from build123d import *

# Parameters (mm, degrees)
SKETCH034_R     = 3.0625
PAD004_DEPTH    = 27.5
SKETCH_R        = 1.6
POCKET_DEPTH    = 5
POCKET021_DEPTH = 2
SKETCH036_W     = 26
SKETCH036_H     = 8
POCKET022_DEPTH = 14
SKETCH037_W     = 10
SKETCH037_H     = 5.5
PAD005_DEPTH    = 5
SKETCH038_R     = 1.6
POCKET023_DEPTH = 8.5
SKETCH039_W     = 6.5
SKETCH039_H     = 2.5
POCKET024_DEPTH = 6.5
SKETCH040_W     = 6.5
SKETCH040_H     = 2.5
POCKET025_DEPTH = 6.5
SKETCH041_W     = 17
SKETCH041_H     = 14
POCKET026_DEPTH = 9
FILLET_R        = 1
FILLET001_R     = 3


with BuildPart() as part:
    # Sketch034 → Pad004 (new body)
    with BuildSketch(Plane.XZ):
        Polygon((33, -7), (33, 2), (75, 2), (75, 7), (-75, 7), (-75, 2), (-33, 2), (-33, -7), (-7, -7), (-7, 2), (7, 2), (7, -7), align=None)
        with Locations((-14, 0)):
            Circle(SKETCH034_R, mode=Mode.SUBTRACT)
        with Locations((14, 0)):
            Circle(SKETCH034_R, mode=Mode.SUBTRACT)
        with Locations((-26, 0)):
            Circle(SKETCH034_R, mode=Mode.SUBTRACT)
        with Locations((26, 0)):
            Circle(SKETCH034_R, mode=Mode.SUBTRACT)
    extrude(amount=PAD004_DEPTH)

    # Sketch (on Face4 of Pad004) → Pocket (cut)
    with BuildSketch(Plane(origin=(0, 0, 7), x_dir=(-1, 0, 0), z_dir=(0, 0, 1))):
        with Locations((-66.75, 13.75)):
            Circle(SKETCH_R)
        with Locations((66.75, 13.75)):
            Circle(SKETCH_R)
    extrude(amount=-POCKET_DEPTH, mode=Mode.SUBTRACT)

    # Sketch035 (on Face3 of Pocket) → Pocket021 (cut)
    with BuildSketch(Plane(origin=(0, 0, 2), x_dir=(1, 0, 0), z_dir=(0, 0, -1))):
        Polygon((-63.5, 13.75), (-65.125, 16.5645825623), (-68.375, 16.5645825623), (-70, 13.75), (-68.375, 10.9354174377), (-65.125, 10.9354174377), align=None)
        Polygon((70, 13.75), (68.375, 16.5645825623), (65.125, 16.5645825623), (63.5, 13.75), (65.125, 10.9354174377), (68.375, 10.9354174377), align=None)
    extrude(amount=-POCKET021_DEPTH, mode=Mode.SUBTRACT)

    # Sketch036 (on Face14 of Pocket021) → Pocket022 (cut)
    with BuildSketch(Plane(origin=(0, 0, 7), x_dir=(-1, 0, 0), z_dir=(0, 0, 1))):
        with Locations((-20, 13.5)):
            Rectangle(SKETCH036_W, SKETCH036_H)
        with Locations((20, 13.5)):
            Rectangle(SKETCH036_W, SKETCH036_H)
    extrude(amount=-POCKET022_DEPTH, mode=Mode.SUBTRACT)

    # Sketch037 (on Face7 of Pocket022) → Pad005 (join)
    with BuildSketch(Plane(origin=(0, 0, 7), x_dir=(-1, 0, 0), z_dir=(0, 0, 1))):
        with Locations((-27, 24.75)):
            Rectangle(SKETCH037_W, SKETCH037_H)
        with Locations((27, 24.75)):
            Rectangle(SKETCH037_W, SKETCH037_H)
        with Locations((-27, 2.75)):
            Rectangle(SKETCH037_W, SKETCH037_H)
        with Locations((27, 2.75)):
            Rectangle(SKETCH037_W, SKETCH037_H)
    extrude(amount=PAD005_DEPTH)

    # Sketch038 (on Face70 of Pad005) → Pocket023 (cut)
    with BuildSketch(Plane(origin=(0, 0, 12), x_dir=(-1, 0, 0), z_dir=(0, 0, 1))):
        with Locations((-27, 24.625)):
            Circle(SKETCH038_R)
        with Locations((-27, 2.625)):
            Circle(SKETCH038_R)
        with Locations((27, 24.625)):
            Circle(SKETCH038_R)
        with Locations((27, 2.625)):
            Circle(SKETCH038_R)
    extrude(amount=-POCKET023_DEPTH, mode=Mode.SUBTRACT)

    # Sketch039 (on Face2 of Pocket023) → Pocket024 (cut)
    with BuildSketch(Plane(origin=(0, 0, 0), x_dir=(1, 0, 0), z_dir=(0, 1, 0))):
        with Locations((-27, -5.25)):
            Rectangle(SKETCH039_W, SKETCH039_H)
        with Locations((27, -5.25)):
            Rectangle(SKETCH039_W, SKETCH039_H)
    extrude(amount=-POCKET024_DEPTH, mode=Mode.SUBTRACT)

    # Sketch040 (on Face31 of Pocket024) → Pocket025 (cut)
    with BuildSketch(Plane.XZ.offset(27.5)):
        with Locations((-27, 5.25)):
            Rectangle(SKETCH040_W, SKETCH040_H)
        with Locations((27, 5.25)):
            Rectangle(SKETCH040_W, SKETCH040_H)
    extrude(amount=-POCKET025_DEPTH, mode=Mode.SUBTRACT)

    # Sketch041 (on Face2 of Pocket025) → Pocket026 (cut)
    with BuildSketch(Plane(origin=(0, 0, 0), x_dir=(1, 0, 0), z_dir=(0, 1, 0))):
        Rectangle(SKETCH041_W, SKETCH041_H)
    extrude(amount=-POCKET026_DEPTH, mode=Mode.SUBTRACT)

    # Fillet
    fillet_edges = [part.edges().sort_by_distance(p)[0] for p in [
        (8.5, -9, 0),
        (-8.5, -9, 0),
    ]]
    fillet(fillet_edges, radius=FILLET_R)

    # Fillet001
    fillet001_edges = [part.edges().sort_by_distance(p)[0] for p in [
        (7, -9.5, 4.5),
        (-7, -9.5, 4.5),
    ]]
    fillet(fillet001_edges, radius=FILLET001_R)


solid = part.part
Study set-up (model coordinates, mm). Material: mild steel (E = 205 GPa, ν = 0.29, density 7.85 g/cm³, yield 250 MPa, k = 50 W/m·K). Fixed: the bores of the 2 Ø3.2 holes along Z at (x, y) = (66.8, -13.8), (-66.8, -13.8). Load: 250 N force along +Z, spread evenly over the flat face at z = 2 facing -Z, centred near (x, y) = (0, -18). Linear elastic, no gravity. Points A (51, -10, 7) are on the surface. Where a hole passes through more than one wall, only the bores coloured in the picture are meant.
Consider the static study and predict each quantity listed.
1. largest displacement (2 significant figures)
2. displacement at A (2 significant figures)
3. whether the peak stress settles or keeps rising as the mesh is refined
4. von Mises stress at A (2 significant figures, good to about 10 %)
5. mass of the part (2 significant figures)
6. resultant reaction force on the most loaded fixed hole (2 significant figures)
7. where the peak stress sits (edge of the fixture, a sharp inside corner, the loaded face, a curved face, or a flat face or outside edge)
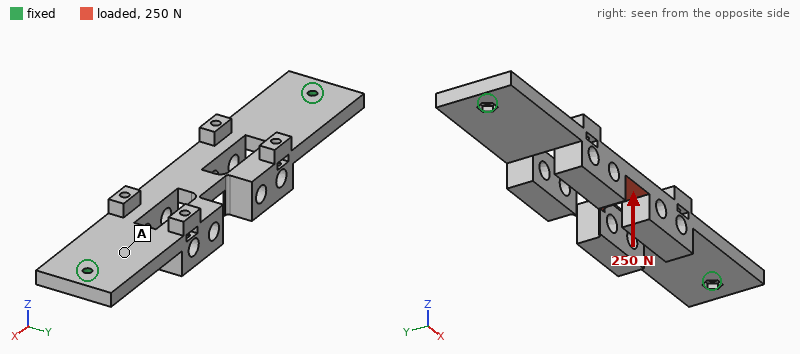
86 µm
16 µm
keeps rising
14 MPa
190 g
230 N
edge of the fixture
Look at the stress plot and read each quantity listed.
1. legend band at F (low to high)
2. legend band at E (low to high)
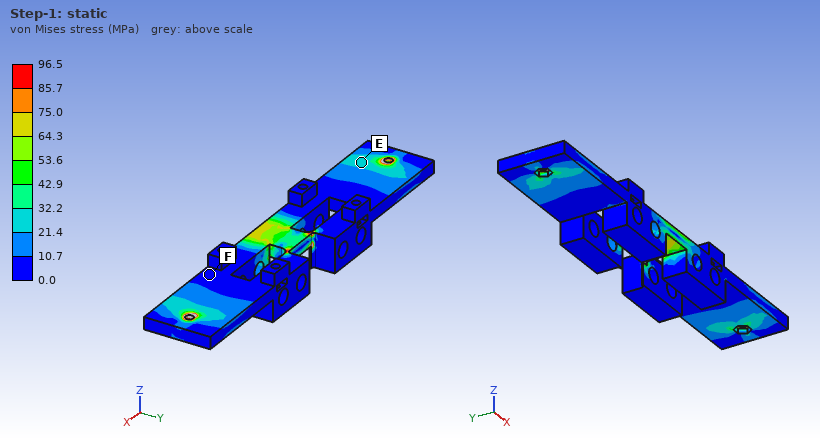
0.0 to 10.7 MPa
21.4 to 32.2 MPa
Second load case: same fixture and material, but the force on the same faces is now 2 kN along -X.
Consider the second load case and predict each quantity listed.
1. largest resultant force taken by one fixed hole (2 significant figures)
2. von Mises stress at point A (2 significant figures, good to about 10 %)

1.0 kN
8.2 MPa
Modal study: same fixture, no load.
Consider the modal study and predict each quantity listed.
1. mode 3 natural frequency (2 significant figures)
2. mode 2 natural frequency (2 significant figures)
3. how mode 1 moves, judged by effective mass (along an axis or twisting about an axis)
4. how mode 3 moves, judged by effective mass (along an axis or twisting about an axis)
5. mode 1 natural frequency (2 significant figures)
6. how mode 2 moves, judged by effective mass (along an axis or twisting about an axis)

2700 Hz
2000 Hz
along Z
along Y
1000 Hz
along Y
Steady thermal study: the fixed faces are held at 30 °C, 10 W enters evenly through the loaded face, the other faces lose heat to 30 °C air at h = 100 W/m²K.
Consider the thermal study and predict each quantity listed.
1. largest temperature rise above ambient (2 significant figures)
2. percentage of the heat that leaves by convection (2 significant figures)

26 K
88 %
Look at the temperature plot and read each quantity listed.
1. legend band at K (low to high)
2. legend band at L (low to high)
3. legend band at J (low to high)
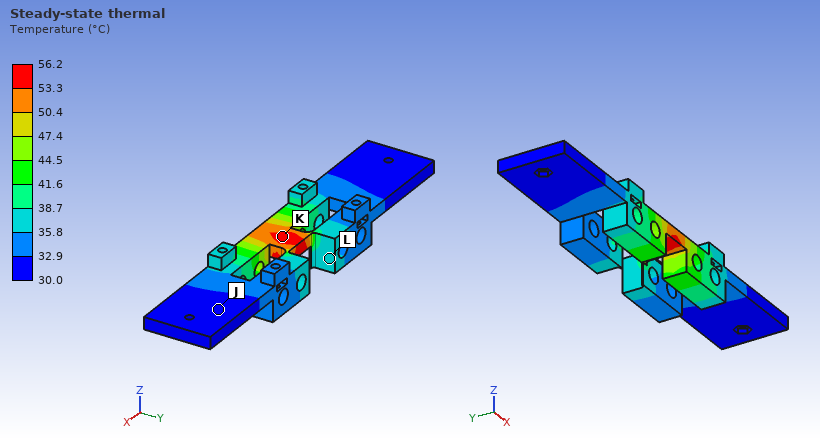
53.3 to 56.2 °C
35.8 to 38.7 °C
30.0 to 32.9 °C
